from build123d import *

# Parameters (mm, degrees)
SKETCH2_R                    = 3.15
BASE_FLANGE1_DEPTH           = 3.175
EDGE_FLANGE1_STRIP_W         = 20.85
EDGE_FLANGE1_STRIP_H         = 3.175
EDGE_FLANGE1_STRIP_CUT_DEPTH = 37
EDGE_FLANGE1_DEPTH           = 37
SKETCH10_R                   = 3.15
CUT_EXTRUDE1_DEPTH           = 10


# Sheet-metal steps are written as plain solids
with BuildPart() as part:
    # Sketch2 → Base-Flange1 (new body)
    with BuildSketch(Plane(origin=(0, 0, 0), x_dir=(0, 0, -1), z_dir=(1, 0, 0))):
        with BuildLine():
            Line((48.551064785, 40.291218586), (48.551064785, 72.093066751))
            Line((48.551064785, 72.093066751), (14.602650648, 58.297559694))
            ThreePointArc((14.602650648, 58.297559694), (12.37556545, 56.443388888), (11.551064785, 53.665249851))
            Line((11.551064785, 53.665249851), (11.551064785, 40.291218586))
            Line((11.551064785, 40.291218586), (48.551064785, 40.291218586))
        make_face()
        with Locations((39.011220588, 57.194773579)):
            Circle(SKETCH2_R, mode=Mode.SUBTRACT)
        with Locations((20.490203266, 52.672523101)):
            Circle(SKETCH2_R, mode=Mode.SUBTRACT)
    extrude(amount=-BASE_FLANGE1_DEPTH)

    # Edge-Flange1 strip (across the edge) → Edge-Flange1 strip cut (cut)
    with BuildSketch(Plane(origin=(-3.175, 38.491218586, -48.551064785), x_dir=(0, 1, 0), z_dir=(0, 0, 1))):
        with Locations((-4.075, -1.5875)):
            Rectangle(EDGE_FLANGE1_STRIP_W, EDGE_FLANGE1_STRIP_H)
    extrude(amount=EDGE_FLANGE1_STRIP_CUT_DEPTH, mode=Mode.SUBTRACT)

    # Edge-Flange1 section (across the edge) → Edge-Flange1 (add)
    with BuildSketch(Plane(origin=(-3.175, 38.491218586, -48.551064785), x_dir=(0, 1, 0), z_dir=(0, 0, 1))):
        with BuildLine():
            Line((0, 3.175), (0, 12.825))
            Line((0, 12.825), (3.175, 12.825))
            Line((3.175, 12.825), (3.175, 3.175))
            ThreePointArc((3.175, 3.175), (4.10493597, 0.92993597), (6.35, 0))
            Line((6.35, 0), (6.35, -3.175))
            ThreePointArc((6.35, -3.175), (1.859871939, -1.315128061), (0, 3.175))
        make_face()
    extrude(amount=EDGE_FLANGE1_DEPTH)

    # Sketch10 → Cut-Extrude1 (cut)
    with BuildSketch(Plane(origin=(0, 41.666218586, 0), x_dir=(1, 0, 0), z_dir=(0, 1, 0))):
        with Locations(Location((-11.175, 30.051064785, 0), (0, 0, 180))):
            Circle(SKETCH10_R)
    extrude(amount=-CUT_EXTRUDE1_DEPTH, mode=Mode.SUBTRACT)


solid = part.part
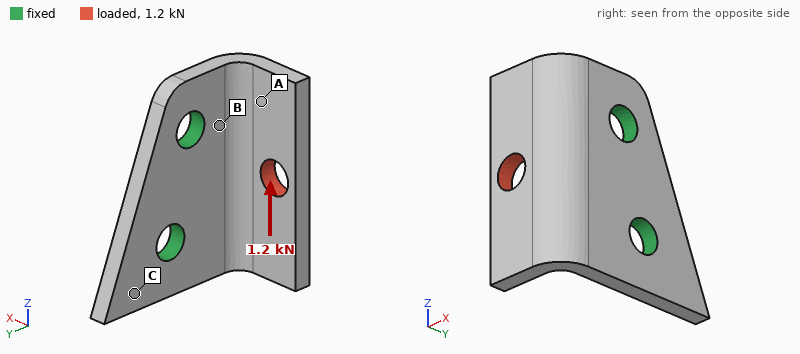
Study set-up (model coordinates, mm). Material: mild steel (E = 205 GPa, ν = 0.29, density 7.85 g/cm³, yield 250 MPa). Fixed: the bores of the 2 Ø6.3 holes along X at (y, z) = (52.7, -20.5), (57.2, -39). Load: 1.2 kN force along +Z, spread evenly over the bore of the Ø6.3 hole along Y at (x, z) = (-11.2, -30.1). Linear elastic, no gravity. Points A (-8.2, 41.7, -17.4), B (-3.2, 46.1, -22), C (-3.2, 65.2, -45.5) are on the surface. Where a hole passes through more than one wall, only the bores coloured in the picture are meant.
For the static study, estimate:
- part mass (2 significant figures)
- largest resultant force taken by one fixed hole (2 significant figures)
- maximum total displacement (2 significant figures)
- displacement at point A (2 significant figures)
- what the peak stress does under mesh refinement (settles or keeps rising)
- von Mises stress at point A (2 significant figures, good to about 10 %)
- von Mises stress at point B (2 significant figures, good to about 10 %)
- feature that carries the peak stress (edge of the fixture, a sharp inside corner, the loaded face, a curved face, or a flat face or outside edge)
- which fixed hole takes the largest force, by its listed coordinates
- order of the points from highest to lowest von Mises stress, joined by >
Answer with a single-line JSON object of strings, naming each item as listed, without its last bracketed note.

{"part mass": "32 g", "largest resultant force taken by one fixed hole": "1.1 kN", "maximum total displacement": "58 µm", "displacement at point A": "18 µm", "what the peak stress does under mesh refinement": "keeps rising", "von Mises stress at point A": "51 MPa", "von Mises stress at point B": "99 MPa", "feature that carries the peak stress": "edge of the fixture", "which fixed hole takes the largest force, by its listed coordinates": "(52.7, -20.5)", "order of the points from highest to lowest von Mises stress, joined by >": "B > A > C"}
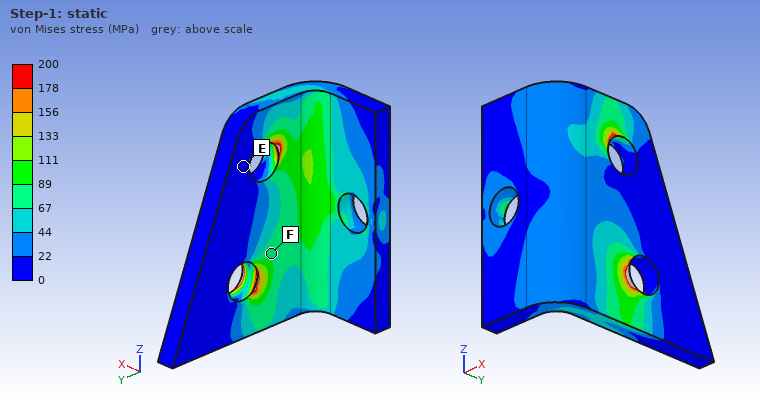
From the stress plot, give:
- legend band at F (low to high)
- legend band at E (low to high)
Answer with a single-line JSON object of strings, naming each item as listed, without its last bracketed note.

{"legend band at F": "67 to 89 MPa", "legend band at E": "0 to 22 MPa"}
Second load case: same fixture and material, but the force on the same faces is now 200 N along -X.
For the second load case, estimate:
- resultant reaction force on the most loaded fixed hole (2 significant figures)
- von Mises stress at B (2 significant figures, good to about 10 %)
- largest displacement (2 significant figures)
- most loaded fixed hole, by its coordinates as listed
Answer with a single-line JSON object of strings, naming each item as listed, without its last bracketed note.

{"resultant reaction force on the most loaded fixed hole": "130 N", "von Mises stress at B": "26 MPa", "largest displacement": "17 µm", "most loaded fixed hole, by its coordinates as listed": "(52.7, -20.5)"}
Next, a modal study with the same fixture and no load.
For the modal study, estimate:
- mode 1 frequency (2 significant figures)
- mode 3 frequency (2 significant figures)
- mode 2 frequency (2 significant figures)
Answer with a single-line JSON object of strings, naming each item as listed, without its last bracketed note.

{"mode 1 frequency": "5000 Hz", "mode 3 frequency": "13 kHz", "mode 2 frequency": "7700 Hz"}
